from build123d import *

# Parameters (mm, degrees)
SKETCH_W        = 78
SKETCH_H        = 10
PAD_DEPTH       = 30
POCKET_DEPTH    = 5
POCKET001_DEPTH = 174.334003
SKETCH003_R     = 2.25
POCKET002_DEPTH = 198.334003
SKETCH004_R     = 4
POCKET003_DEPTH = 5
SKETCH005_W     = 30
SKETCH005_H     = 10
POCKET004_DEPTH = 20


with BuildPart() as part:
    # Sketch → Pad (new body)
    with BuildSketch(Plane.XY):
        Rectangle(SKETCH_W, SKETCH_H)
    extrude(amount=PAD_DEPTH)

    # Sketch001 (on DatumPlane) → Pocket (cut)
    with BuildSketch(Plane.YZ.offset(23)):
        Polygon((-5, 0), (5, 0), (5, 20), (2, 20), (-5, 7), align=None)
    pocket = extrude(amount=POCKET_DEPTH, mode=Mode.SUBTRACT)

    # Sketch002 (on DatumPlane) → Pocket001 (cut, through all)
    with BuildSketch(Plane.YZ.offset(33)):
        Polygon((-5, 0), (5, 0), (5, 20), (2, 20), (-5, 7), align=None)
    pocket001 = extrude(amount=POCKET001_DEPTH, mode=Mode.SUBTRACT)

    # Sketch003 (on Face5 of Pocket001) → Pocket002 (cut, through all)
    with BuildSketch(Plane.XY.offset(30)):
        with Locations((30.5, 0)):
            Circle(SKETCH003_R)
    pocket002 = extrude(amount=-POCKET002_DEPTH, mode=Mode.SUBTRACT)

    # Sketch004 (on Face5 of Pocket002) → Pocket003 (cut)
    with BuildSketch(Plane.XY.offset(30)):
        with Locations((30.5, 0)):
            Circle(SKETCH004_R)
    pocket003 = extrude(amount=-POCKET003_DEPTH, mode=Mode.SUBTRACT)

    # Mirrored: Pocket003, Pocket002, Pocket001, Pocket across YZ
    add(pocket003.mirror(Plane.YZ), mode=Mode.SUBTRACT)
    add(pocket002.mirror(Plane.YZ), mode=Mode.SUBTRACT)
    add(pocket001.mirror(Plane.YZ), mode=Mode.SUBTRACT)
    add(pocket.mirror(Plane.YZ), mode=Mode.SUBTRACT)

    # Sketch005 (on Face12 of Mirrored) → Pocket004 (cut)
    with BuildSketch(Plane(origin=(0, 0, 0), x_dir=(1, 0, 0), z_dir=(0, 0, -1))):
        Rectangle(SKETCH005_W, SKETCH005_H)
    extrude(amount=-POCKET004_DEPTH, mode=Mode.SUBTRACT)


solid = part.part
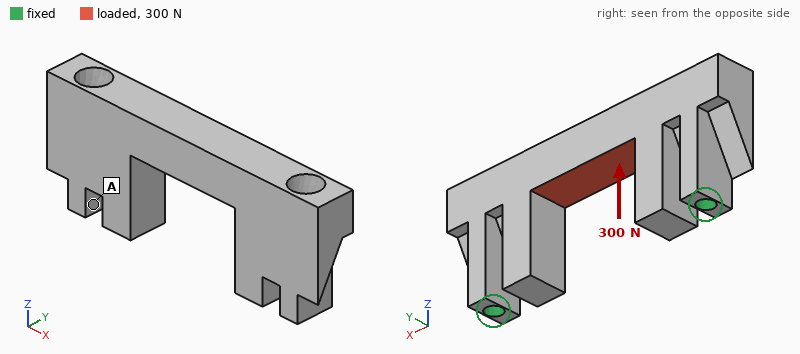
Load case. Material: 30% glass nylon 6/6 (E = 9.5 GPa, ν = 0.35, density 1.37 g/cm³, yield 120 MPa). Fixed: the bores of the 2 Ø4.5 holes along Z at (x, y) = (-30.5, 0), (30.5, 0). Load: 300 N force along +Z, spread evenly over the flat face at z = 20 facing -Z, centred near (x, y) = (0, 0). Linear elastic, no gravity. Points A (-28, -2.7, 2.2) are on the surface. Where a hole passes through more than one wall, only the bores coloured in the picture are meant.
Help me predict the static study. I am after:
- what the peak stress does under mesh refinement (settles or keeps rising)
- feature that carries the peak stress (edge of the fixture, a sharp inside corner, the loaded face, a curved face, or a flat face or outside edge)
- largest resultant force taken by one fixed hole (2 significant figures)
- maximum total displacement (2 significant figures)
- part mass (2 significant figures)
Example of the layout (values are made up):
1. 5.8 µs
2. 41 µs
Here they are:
1. keeps rising
2. edge of the fixture
3. 190 N
4. 30 µm
5. 17 g
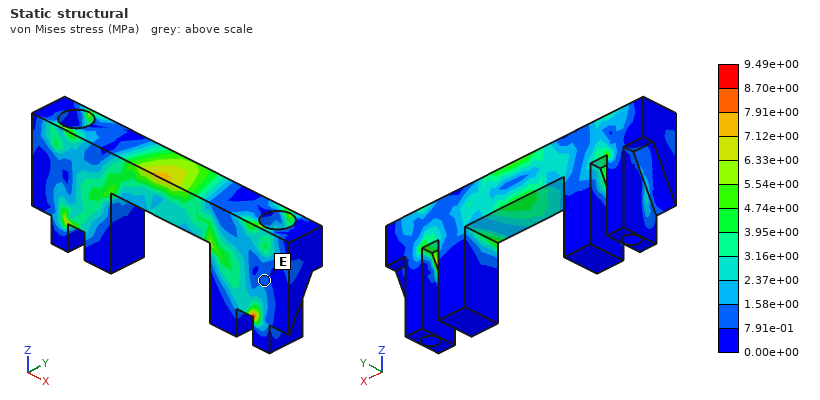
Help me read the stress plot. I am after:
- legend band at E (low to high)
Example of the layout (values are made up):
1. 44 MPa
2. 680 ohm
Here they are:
1. 7.91e-01 to 1.58e+00 MPa
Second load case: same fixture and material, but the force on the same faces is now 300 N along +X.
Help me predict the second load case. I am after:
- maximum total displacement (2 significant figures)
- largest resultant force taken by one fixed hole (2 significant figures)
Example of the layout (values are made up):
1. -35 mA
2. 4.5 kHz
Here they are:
1. 6.6 µm
2. 150 N
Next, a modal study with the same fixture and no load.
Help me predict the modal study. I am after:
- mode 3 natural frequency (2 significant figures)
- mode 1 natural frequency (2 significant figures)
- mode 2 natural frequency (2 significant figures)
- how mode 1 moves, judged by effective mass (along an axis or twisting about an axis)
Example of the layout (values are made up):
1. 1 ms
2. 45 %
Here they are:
1. 6000 Hz
2. 4900 Hz
3. 5900 Hz
4. along Y
